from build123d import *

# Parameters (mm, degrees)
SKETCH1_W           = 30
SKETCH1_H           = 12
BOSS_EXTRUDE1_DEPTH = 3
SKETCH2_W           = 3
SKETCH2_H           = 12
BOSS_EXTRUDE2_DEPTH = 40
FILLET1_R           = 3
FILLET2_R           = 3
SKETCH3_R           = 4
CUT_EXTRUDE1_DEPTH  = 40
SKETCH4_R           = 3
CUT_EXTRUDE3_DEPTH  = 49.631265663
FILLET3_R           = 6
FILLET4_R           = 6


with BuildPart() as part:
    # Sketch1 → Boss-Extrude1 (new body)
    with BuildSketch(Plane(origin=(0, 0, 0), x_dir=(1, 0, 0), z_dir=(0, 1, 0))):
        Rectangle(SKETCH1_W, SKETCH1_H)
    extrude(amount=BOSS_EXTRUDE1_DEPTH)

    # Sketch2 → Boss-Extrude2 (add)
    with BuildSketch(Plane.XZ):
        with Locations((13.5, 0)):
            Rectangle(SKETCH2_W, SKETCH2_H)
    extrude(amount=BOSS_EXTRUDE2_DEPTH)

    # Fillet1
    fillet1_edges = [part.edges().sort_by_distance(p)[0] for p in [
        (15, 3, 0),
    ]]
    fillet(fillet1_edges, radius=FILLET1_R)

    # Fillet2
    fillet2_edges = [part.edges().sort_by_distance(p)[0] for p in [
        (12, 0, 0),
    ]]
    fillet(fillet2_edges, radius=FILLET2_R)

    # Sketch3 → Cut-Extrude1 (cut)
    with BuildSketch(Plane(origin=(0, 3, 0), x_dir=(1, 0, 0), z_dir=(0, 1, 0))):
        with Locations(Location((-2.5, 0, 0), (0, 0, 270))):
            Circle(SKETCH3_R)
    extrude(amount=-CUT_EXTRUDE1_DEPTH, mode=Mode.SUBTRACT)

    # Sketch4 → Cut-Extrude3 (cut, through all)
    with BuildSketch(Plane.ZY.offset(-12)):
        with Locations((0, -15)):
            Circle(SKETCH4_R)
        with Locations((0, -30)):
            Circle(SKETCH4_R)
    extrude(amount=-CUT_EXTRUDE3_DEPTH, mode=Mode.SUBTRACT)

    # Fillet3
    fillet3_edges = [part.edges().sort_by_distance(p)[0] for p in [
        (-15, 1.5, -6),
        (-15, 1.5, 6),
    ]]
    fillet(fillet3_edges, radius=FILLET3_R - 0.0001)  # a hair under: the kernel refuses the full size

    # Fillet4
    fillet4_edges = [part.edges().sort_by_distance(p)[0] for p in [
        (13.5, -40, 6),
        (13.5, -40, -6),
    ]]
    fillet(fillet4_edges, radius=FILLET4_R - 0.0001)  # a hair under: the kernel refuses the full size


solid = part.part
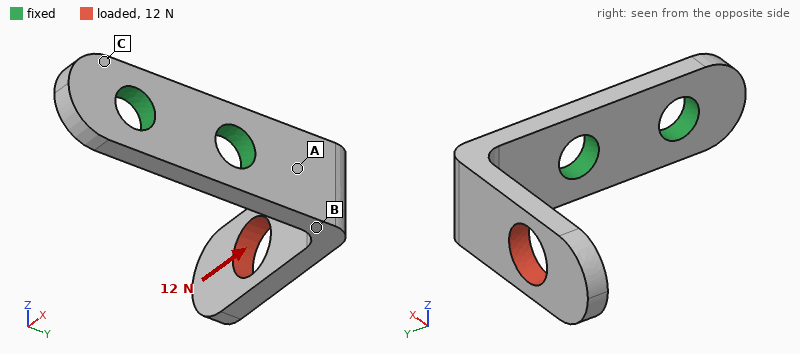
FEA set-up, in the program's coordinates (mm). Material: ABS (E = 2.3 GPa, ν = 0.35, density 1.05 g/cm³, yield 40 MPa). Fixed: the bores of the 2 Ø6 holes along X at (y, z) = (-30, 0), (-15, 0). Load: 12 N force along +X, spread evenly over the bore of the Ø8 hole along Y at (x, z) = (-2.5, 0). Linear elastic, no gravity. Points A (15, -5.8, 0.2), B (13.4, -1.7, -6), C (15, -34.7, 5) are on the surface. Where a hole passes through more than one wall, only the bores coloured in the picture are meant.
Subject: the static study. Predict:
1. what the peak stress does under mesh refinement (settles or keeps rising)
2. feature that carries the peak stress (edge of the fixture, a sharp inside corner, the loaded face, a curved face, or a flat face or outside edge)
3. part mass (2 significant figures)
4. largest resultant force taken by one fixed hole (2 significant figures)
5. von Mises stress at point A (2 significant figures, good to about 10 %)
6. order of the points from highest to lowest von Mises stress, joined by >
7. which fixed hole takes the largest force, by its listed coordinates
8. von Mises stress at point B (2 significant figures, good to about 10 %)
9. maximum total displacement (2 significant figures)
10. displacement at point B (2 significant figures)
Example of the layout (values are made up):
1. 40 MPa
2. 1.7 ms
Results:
1. keeps rising
2. edge of the fixture
3. 2.2 g
4. 12 N
5. 4.4 MPa
6. A > B > C
7. (-15, 0)
8. 1.9 MPa
9. 0.58 mm
10. 0.13 mm
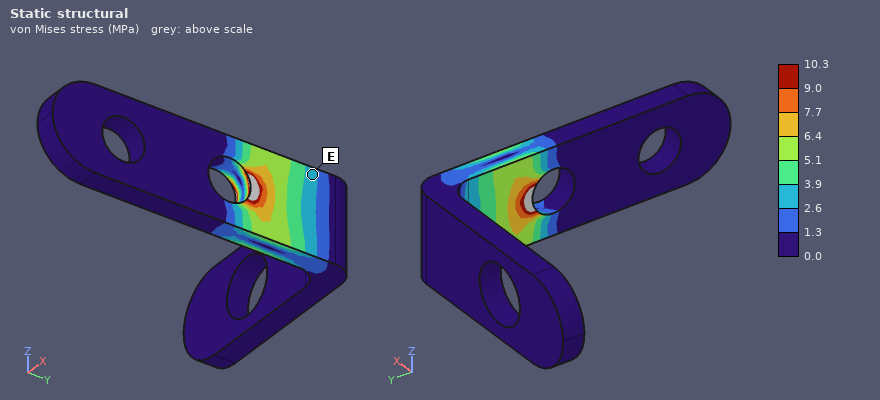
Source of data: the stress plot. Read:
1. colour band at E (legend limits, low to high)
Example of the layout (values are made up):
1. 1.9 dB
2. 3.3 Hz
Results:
1. 2.6 to 3.9 MPa
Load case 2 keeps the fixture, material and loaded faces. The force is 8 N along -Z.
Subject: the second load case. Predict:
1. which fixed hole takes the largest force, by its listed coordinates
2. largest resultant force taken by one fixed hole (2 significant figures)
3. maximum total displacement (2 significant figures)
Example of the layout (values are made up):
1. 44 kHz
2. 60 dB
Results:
1. (-15, 0)
2. 9.6 N
3. 0.52 mm
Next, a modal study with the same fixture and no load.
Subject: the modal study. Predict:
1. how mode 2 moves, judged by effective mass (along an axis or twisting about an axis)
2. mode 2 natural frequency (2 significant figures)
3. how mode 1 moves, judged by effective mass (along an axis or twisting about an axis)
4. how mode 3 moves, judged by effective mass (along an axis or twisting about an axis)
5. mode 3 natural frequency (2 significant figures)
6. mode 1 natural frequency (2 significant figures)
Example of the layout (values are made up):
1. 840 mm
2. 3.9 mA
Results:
1. along Z
2. 880 Hz
3. along Y
4. along X
5. 1900 Hz
6. 590 Hz
